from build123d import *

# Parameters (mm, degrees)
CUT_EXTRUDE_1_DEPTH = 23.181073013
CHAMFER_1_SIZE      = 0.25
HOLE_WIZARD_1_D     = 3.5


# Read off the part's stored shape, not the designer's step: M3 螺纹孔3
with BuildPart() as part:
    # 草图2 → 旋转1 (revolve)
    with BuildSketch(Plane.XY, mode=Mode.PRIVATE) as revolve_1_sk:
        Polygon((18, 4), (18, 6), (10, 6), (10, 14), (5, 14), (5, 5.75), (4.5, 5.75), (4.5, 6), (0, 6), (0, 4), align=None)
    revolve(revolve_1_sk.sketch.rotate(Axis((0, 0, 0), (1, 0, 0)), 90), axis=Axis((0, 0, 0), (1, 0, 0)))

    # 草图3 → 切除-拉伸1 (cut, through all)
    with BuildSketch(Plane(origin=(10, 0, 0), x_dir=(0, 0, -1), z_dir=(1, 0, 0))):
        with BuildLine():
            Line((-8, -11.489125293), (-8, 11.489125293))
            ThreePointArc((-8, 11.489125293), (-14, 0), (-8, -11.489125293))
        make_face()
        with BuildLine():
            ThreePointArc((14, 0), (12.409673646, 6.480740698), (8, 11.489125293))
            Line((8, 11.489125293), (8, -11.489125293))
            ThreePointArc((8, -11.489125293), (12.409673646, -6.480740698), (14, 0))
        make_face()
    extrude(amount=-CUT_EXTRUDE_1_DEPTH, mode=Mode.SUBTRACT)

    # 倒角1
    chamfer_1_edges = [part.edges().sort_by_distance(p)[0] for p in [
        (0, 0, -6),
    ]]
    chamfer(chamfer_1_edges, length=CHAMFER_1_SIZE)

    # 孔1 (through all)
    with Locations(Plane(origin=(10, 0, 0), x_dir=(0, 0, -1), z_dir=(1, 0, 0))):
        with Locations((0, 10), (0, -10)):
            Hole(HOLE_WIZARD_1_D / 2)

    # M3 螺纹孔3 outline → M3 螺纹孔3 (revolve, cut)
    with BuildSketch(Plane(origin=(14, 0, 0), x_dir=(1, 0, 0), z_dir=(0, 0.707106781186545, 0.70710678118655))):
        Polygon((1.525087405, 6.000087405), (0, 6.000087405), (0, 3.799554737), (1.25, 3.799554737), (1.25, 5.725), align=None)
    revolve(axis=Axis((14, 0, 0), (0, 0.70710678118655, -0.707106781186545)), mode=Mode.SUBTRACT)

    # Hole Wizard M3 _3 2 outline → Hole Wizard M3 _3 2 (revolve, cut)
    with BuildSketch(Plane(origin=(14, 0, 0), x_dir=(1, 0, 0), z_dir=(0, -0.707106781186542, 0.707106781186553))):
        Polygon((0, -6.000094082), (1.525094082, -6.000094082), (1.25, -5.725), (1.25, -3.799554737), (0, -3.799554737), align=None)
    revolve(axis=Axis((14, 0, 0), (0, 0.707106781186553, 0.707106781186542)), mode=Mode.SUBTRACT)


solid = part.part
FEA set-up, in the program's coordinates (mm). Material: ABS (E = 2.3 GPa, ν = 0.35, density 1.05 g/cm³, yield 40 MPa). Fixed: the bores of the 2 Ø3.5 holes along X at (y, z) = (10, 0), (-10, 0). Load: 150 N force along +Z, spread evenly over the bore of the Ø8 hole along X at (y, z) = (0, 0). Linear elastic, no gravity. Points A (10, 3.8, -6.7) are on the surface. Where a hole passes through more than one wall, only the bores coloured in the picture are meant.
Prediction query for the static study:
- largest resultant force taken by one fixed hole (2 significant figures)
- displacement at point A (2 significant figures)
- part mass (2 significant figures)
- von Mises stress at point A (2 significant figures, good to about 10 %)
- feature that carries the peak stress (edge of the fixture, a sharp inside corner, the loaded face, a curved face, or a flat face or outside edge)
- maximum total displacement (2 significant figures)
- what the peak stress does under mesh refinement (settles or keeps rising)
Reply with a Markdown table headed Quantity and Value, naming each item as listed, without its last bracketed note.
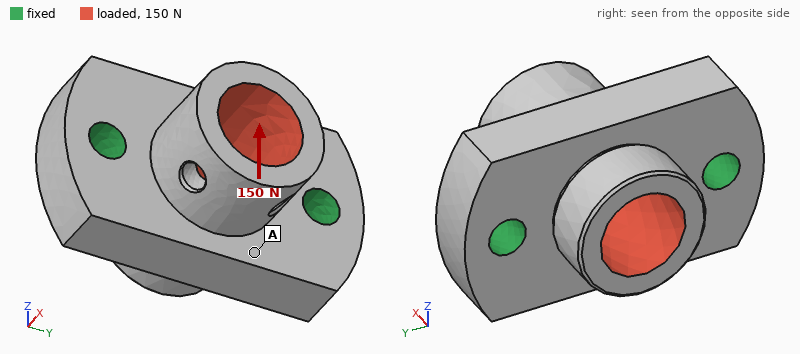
| Quantity | Value |
|---|---|
| largest resultant force taken by one fixed hole | 75 N |
| displacement at point A | 14 µm |
| part mass | 2.7 g |
| von Mises stress at point A | 1.3 MPa |
| feature that carries the peak stress | edge of the fixture |
| maximum total displacement | 41 µm |
| what the peak stress does under mesh refinement | keeps rising |
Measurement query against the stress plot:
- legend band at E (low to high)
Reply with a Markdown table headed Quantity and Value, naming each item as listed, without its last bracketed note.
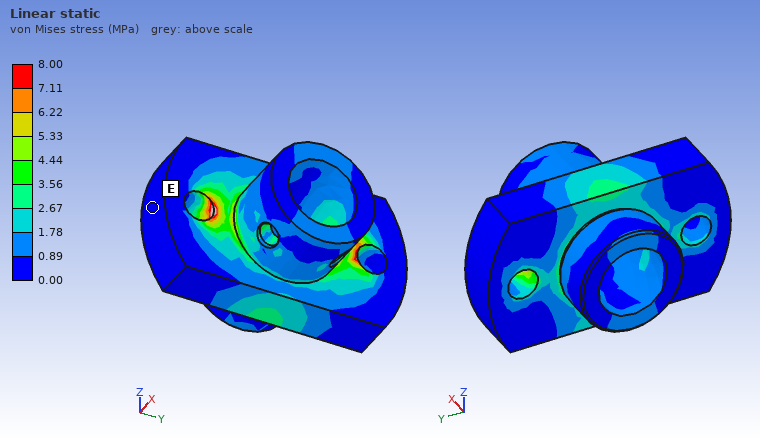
| Quantity | Value |
|---|---|
| legend band at E | 0.00 to 0.89 MPa |
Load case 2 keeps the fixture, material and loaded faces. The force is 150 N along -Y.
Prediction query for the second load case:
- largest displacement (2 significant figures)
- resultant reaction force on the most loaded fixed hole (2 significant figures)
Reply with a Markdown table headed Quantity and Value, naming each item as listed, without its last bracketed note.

| Quantity | Value |
|---|---|
| largest displacement | 22 µm |
| resultant reaction force on the most loaded fixed hole | 76 N |
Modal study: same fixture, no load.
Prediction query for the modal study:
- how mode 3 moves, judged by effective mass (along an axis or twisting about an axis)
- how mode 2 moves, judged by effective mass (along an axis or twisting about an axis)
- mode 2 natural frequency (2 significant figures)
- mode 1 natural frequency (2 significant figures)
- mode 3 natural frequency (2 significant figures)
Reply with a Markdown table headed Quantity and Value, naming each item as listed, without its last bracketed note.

| Quantity | Value |
|---|---|
| how mode 3 moves, judged by effective mass | along Y |
| how mode 2 moves, judged by effective mass | along X |
| mode 2 natural frequency | 11 kHz |
| mode 1 natural frequency | 7200 Hz |
| mode 3 natural frequency | 13 kHz |
